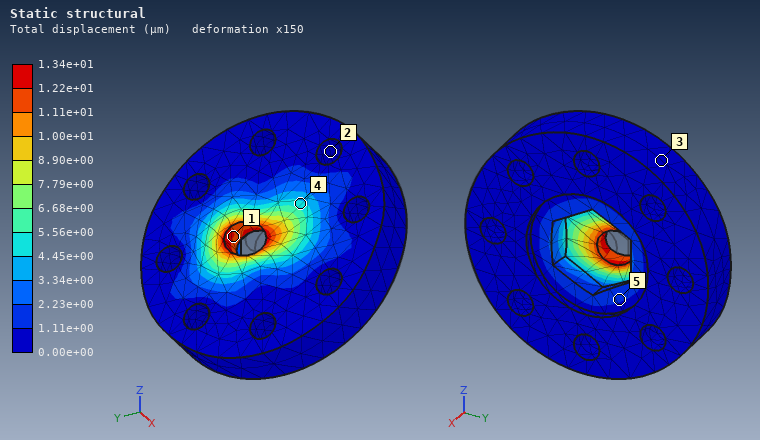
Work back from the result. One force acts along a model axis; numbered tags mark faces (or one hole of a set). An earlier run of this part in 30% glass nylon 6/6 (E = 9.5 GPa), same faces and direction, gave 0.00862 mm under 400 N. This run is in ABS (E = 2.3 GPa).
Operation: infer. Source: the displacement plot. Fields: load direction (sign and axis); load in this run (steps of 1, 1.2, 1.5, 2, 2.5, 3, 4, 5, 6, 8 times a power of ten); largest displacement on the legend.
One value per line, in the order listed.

+Y
150 N
1.34e+01 µm
